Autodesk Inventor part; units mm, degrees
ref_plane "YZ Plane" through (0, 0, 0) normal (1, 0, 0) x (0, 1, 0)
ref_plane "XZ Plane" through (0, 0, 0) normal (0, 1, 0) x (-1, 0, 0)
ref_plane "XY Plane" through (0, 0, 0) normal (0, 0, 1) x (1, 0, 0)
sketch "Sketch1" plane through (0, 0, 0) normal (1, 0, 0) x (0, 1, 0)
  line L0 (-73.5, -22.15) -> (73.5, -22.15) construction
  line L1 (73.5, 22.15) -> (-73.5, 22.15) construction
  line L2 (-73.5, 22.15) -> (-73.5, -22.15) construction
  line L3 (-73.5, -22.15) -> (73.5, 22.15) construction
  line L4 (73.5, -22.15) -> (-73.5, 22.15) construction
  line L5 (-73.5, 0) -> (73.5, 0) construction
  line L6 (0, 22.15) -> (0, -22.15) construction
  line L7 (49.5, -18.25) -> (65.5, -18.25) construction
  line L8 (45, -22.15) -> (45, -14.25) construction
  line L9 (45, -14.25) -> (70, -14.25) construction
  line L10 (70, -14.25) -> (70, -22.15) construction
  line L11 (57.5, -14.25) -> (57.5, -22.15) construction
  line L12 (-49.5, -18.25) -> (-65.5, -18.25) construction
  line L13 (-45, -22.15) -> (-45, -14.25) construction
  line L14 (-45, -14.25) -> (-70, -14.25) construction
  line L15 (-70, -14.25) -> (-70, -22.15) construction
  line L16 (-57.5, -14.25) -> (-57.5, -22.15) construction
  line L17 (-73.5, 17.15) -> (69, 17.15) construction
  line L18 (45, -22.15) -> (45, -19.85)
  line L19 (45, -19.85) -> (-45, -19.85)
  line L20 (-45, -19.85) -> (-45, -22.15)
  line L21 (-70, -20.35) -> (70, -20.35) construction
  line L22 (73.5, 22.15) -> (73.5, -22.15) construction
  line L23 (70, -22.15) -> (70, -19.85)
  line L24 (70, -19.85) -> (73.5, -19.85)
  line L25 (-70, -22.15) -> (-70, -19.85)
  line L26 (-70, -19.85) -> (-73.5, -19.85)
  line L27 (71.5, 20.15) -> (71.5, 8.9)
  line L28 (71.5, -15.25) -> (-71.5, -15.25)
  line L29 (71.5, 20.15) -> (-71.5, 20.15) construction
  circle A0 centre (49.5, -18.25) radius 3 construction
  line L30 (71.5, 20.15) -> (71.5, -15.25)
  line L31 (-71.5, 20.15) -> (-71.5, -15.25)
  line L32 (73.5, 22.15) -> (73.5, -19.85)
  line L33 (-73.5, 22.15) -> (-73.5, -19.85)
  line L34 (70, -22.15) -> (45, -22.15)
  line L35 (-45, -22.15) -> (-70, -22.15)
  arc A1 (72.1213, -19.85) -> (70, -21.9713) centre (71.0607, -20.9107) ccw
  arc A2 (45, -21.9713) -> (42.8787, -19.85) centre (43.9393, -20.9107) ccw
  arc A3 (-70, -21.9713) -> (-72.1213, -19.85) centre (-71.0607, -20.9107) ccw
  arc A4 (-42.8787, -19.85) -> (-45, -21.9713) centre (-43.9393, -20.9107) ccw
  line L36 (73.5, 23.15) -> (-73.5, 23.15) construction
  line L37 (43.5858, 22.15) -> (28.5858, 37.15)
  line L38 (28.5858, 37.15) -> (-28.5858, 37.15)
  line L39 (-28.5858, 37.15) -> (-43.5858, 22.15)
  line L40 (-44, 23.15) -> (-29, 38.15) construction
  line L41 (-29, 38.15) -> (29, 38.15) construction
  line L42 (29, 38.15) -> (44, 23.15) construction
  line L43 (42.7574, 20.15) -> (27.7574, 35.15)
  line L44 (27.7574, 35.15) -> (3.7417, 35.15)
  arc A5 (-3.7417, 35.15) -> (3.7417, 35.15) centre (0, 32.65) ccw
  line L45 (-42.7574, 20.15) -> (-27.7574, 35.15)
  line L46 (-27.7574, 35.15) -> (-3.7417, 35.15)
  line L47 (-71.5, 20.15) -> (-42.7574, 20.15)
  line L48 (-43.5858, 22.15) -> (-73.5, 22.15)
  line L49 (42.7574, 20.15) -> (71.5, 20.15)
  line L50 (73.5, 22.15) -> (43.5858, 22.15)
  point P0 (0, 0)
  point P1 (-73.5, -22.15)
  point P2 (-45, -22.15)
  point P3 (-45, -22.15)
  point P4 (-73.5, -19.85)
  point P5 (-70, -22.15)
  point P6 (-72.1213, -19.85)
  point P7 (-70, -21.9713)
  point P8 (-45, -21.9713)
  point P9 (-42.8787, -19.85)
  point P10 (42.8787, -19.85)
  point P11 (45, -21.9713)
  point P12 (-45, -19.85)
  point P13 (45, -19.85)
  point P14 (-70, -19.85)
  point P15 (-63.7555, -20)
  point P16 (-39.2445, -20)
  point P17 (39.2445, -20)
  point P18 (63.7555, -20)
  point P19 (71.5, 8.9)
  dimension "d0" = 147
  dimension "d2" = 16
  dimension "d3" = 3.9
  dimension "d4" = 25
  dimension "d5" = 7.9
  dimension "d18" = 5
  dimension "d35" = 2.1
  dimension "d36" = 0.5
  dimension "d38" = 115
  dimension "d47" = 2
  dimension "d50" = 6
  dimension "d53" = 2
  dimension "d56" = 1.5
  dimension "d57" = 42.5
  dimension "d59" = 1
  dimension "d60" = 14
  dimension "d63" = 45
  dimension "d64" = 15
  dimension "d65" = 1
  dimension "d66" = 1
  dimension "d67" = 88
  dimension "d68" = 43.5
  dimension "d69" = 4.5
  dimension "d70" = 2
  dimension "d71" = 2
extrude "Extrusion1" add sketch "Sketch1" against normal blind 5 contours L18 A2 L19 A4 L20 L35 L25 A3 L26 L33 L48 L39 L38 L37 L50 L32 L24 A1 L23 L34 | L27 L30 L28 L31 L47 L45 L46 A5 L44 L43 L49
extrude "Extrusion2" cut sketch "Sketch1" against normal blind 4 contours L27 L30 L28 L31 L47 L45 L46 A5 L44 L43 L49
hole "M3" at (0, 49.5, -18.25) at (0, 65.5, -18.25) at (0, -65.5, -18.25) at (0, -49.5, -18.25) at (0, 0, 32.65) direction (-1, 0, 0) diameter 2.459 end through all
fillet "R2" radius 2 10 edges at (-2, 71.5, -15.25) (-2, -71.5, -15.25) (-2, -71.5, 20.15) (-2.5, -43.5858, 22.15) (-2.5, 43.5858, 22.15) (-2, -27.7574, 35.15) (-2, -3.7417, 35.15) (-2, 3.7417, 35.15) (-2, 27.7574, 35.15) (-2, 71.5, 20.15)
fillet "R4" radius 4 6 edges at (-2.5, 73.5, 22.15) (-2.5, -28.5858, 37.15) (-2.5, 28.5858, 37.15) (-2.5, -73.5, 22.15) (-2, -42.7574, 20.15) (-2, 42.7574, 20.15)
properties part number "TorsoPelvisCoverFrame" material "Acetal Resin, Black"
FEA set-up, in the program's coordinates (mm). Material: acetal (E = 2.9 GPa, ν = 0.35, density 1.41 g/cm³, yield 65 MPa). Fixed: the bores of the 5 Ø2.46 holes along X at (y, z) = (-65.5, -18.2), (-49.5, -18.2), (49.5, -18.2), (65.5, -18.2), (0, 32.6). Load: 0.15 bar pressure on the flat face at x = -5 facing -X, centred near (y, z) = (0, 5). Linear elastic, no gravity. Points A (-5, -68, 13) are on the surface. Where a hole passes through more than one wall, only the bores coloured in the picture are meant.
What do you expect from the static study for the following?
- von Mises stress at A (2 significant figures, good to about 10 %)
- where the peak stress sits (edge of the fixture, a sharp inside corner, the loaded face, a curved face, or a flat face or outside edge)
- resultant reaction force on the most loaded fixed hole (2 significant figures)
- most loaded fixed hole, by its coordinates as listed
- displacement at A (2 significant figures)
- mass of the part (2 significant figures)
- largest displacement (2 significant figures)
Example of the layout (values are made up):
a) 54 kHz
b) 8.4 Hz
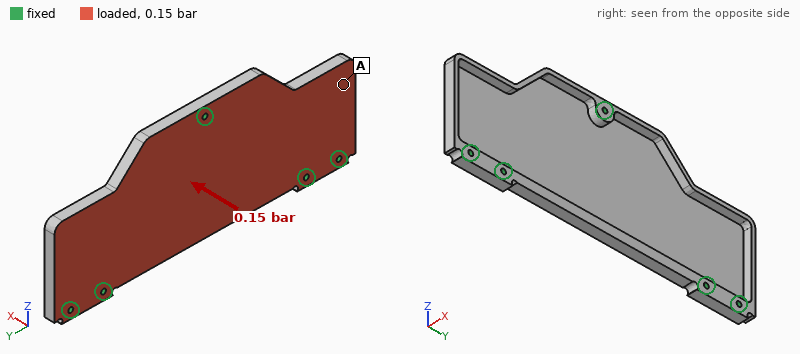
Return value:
a) 2.9 MPa
b) the loaded face
c) 57 N
d) (0, 32.6)
e) 0.86 mm
f) 18 g
g) 1.4 mm
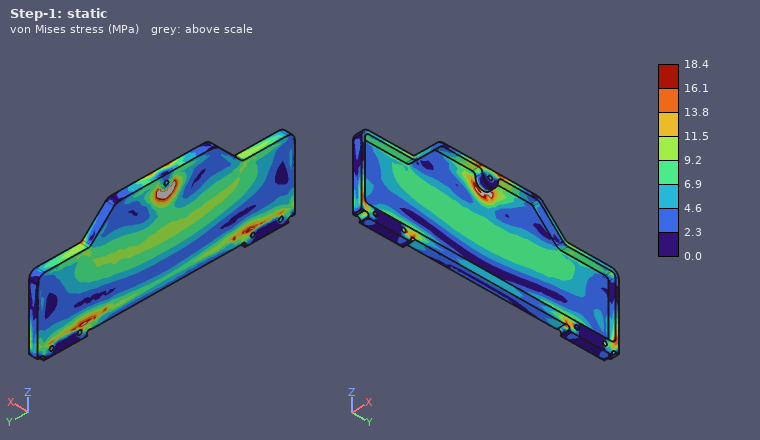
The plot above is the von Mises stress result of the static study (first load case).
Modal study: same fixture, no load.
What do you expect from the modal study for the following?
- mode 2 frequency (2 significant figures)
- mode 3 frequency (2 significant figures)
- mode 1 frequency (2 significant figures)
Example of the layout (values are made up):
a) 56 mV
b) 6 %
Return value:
a) 450 Hz
b) 570 Hz
c) 450 Hz
